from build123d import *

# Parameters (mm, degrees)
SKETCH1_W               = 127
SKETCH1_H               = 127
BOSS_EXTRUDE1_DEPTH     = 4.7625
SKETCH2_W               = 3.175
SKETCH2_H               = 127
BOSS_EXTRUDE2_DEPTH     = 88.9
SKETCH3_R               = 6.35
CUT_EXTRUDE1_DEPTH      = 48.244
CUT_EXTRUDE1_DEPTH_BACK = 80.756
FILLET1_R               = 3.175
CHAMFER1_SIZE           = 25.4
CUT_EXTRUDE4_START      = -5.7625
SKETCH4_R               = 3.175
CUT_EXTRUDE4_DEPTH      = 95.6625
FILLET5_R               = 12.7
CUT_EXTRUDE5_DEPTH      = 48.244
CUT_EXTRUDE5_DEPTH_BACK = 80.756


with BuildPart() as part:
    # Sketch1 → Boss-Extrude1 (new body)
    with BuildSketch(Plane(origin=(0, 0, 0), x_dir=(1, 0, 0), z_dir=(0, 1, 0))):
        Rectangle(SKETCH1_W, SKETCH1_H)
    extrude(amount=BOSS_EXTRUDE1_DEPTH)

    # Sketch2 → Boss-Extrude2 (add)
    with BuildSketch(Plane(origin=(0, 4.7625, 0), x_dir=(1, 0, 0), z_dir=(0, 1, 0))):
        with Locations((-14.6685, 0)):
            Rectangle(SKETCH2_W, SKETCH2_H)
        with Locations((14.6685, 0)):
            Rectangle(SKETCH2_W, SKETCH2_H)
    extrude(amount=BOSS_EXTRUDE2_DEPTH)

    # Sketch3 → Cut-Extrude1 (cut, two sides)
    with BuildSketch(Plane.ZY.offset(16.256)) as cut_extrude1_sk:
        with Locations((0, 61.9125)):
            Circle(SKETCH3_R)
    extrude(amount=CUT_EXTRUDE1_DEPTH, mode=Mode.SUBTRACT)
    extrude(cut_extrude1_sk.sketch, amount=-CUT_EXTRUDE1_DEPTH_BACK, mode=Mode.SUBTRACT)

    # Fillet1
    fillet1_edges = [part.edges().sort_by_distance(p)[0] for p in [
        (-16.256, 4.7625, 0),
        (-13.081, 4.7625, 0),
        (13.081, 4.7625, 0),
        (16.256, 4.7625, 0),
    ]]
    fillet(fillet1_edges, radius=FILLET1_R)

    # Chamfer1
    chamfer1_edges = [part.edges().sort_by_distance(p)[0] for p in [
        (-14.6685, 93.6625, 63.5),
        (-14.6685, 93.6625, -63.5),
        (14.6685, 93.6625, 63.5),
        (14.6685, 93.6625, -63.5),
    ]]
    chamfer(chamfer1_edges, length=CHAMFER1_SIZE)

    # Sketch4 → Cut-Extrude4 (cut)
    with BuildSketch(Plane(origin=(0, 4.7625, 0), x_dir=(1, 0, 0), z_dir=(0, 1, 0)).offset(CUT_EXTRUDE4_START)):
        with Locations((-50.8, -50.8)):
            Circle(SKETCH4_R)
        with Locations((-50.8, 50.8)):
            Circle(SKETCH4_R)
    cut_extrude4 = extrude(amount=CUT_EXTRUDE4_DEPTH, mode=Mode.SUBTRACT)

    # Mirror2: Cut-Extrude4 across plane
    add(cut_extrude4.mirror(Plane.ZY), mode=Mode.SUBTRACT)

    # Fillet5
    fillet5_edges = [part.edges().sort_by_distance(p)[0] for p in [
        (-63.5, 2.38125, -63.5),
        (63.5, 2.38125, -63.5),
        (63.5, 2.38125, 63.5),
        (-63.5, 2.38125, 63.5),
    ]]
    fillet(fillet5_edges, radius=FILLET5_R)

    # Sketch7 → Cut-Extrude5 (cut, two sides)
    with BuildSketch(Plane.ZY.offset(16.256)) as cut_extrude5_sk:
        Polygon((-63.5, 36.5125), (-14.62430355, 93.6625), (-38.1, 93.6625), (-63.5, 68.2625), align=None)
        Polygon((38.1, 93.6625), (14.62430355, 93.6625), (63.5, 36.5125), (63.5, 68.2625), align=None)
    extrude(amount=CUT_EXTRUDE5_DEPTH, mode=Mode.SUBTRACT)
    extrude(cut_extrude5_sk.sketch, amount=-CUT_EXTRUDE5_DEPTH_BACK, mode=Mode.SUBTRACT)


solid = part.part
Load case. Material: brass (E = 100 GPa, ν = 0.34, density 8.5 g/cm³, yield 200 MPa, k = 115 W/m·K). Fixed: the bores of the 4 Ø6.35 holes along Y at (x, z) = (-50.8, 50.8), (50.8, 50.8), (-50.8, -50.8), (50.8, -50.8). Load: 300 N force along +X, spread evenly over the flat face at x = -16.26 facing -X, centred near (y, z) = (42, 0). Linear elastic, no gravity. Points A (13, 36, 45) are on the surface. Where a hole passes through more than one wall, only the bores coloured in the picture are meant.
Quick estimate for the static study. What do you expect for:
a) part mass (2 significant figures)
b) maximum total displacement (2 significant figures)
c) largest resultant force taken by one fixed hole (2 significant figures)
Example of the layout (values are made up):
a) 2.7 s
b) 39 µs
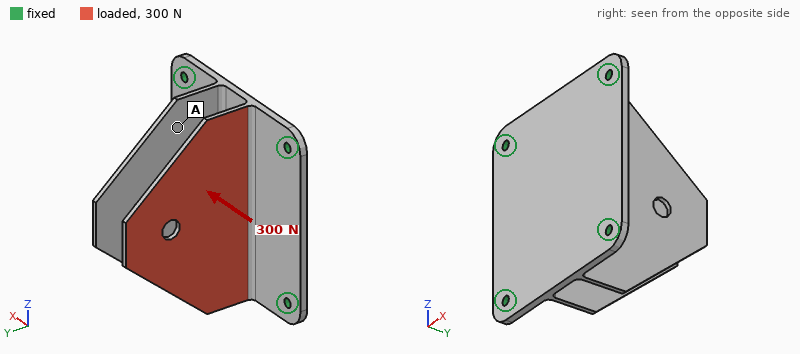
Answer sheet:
a) 1.1 kg
b) 0.63 mm
c) 110 N
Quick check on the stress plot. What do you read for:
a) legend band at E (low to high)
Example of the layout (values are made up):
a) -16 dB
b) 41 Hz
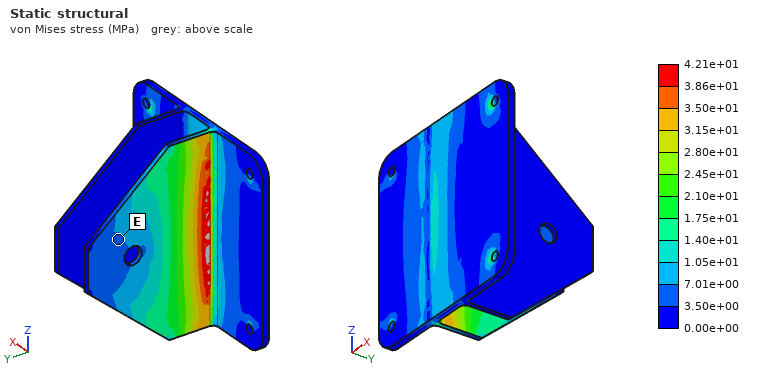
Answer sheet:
a) 3.50e+00 to 7.01e+00 MPa
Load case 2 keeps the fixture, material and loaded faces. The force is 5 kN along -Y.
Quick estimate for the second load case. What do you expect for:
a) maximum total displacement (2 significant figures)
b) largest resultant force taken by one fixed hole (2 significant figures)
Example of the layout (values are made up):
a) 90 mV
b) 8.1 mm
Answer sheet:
a) 0.50 mm
b) 1.8 kN
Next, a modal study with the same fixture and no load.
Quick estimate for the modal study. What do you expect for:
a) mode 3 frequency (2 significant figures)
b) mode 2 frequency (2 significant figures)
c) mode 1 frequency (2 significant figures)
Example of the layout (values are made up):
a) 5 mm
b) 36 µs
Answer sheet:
a) 780 Hz
b) 330 Hz
c) 310 Hz
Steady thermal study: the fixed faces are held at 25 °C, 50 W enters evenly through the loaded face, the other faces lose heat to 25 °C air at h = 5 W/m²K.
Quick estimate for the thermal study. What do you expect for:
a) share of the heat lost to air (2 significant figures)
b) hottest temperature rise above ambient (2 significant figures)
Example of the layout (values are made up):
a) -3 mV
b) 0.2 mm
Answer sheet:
a) 11 %
b) 69 K
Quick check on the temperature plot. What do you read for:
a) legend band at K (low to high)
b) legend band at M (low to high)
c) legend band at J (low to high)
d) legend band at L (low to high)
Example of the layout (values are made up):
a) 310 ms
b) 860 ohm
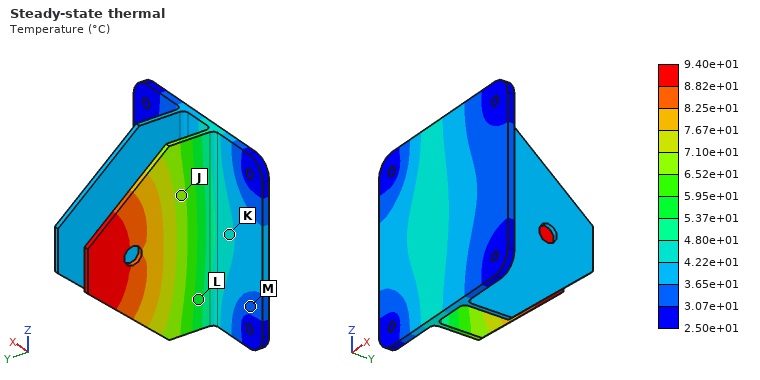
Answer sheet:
a) 4.22e+01 to 4.80e+01 °C
b) 3.07e+01 to 3.65e+01 °C
c) 6.52e+01 to 7.10e+01 °C
d) 5.37e+01 to 5.95e+01 °C
